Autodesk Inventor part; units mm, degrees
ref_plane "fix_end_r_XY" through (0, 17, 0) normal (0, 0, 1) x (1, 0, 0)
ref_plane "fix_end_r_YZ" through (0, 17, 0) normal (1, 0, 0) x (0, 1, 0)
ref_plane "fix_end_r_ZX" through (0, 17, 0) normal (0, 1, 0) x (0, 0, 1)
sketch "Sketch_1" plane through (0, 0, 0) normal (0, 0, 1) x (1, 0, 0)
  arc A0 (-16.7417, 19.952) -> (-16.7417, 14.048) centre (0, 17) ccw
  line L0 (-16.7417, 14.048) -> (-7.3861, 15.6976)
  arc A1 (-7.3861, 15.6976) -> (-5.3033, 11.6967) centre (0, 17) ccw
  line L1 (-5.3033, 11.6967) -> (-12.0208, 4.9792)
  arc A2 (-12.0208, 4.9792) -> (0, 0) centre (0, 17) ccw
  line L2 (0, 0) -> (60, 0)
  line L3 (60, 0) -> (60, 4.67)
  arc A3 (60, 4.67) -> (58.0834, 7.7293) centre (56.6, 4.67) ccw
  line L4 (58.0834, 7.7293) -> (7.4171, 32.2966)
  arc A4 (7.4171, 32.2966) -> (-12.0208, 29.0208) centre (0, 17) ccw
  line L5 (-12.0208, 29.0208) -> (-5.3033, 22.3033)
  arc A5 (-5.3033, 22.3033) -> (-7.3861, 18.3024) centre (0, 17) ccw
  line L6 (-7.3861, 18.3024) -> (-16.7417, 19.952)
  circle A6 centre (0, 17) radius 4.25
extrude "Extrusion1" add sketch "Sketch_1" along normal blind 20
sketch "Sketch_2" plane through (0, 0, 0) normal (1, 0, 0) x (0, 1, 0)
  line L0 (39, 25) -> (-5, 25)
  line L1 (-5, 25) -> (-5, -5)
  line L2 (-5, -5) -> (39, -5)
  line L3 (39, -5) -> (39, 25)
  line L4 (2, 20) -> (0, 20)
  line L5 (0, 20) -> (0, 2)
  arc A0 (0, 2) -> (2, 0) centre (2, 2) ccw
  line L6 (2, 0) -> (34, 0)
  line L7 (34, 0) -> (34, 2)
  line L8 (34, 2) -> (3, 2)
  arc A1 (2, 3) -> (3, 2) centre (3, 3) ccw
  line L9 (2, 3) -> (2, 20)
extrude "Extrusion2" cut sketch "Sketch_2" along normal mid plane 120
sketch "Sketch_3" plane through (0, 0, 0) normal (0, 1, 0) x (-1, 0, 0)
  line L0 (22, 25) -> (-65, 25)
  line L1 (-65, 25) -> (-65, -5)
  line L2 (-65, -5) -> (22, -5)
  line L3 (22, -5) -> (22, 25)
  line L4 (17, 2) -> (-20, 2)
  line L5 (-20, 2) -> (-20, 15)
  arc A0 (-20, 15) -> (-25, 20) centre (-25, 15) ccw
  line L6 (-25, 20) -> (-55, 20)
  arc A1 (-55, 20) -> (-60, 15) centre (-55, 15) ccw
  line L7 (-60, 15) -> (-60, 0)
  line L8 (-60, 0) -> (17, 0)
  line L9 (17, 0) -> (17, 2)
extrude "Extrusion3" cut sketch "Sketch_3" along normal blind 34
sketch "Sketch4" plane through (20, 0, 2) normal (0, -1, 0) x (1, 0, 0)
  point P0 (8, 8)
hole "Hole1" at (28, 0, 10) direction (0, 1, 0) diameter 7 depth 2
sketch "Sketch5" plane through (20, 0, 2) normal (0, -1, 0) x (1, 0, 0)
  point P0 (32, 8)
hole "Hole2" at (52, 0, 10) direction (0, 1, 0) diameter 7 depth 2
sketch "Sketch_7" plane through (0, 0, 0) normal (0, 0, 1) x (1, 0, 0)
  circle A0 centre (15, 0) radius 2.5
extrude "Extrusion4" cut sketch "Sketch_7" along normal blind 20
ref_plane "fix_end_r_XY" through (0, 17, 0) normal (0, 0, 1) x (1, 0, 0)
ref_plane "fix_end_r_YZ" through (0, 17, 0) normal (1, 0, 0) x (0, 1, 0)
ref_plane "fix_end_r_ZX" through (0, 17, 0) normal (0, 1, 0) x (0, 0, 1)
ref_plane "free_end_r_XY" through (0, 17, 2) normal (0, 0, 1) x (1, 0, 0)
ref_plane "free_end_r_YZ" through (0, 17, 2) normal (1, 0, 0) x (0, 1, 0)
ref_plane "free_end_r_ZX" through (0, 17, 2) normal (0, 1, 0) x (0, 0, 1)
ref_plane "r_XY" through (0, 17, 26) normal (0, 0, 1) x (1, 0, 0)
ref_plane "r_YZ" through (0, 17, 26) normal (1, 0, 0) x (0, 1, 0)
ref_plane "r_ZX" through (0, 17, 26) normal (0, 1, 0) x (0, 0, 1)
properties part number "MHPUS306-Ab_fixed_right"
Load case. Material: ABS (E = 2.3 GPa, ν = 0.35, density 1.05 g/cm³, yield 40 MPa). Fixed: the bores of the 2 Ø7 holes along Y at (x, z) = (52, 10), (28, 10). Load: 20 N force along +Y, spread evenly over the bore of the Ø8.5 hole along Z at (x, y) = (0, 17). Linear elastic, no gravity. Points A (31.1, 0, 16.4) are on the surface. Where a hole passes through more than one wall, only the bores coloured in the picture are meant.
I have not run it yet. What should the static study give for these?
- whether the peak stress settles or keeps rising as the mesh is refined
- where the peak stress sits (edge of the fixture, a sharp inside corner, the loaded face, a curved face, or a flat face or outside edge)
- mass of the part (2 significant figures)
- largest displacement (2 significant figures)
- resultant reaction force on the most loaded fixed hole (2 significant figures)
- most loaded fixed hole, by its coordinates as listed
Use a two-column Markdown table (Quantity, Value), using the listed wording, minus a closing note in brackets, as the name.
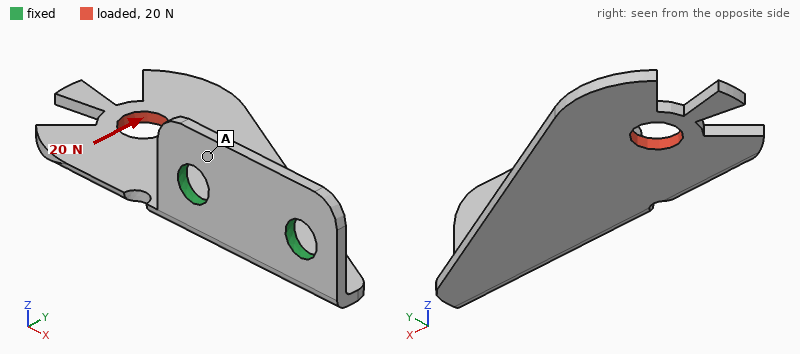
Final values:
| Quantity | Value |
|---|---|
| whether the peak stress settles or keeps rising as the mesh is refined | keeps rising |
| where the peak stress sits | edge of the fixture |
| mass of the part | 4.5 g |
| largest displacement | 1.0 mm |
| resultant reaction force on the most loaded fixed hole | 41 N |
| most loaded fixed hole, by its coordinates as listed | (28, 10) |
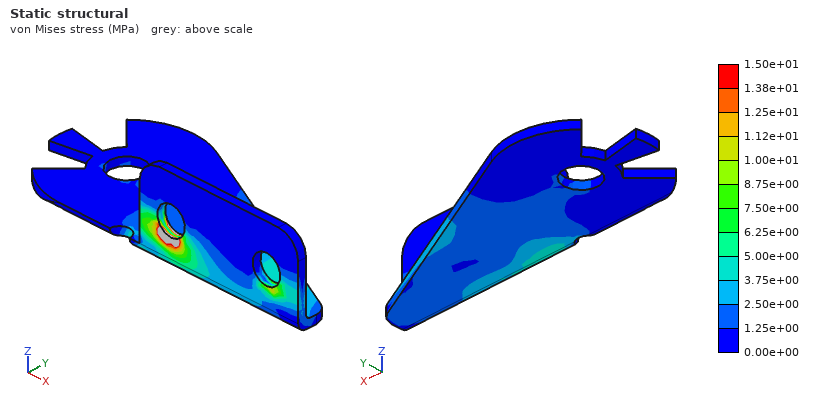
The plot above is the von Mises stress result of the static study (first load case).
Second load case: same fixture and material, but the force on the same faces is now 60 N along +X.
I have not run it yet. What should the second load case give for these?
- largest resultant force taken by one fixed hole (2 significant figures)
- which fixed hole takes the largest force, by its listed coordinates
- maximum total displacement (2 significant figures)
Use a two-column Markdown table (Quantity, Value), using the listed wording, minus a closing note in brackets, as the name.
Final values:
| Quantity | Value |
|---|---|
| largest resultant force taken by one fixed hole | 53 N |
| which fixed hole takes the largest force, by its listed coordinates | (52, 10) |
| maximum total displacement | 0.92 mm |
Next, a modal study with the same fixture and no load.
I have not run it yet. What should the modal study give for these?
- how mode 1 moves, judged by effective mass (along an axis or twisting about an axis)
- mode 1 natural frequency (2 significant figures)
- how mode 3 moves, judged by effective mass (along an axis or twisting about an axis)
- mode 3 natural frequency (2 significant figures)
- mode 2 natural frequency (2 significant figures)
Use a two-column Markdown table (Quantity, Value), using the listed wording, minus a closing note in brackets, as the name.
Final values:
| Quantity | Value |
|---|---|
| how mode 1 moves, judged by effective mass | along Z |
| mode 1 natural frequency | 230 Hz |
| how mode 3 moves, judged by effective mass | along Y |
| mode 3 natural frequency | 880 Hz |
| mode 2 natural frequency | 580 Hz |
